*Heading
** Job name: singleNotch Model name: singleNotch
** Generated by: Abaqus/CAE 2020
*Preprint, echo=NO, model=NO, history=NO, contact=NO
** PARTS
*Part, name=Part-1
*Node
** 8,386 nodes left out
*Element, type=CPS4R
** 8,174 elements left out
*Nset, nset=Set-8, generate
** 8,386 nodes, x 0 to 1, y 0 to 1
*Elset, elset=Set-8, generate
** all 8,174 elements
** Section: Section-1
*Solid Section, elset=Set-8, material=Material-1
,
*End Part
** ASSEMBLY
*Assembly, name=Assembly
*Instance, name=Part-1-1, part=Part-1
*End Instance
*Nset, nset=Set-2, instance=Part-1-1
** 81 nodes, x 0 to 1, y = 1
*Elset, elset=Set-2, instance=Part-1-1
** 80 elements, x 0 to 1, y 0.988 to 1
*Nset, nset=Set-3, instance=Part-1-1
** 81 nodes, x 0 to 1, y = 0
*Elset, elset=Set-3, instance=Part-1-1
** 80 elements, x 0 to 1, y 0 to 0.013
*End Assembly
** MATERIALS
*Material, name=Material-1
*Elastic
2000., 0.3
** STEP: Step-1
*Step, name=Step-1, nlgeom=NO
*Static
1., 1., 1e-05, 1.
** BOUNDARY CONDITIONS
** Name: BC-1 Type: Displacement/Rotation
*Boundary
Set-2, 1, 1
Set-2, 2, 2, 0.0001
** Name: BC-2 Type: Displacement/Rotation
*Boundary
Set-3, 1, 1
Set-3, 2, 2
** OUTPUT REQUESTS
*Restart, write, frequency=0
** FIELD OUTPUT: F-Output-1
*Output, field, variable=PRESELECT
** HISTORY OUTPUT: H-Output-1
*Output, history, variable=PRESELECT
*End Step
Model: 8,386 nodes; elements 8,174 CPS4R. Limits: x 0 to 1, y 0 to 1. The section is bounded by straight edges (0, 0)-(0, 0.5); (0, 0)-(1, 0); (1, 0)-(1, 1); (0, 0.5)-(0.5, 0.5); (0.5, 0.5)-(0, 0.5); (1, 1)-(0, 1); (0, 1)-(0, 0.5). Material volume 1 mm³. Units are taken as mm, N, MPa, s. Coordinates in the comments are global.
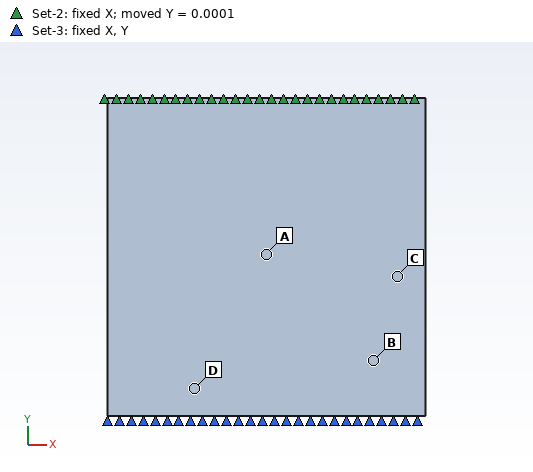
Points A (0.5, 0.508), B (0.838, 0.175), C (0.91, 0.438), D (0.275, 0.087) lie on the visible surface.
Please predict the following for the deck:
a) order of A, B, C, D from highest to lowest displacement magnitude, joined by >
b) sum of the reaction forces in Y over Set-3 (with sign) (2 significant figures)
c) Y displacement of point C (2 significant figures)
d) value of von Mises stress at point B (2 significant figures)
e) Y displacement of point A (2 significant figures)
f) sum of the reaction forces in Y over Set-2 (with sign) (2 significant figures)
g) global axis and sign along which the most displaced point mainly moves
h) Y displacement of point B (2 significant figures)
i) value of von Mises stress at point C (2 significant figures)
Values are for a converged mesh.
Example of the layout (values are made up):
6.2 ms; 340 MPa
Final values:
A > C > B > D; -0.12 N; 4.4e-05 mm; 0.21 MPa; 5.5e-05 mm; 0.12 N; +Y; 1.7e-05 mm; 0.18 MPa
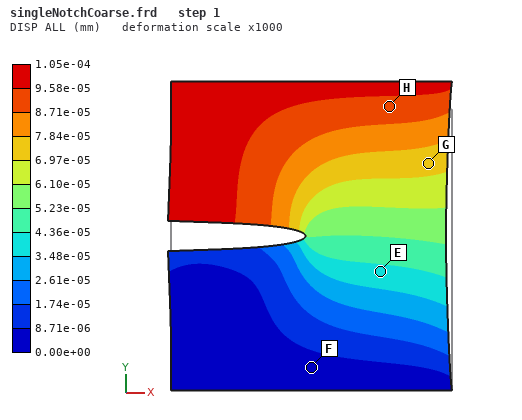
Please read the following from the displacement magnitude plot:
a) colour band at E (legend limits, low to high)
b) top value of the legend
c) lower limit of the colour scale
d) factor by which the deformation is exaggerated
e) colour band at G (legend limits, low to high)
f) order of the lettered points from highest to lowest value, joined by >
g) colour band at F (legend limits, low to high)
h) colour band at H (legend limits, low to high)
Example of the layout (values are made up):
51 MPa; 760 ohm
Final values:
3.48e-05 to 4.36e-05 mm; 1.05e-04 mm; 0.00e+00 mm; 1000; 6.97e-05 to 7.84e-05 mm; H > G > E > F; 0.00e+00 to 8.71e-06 mm; 8.71e-05 to 9.58e-05 mm
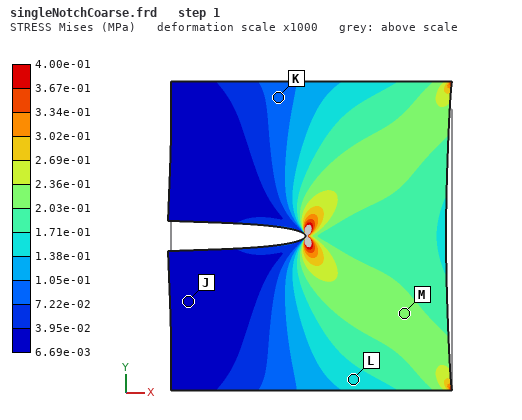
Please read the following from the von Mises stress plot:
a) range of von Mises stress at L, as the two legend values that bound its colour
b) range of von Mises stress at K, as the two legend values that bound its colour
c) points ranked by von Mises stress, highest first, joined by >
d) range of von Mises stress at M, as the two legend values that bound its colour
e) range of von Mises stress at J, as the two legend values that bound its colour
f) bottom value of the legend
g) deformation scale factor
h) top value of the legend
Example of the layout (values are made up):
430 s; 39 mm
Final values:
1.38e-01 to 1.71e-01 MPa; 7.22e-02 to 1.05e-01 MPa; M > L > K > J; 2.03e-01 to 2.36e-01 MPa; 6.69e-03 to 3.95e-02 MPa; 6.69e-03 MPa; 1000; 4.00e-01 MPa
